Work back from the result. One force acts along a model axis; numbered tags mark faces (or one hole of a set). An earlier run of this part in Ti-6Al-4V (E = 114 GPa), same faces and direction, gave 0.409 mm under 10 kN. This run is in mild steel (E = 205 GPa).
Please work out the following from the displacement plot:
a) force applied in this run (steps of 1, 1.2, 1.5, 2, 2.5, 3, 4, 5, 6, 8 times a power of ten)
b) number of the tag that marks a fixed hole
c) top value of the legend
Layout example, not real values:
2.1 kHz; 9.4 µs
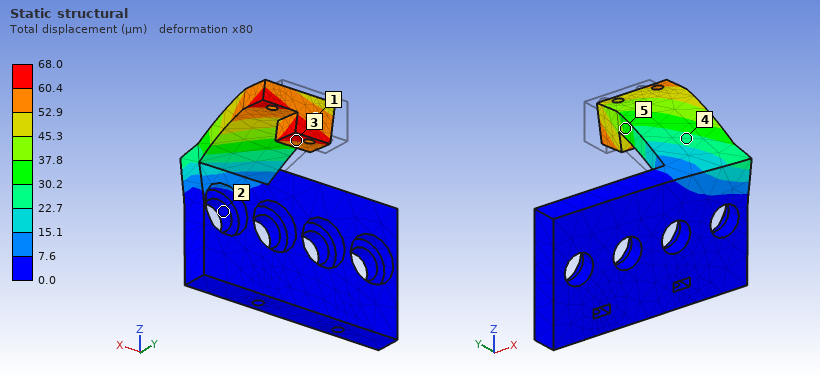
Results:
3 kN; 2; 68.0 µm
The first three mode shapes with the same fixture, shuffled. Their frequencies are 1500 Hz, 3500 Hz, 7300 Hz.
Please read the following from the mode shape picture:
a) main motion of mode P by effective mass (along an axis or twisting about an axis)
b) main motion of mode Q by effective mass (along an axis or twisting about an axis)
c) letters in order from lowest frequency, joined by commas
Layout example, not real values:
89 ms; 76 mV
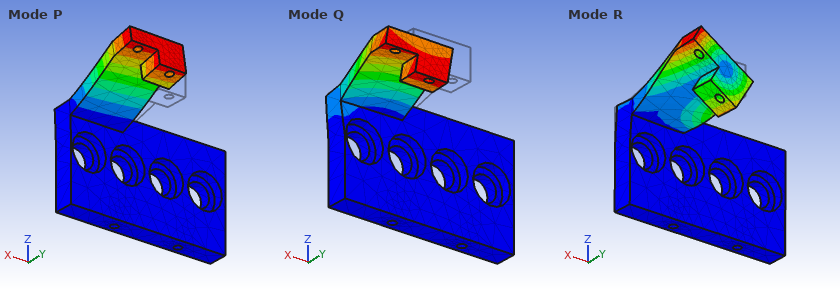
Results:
along Z; along X; P, Q, R
